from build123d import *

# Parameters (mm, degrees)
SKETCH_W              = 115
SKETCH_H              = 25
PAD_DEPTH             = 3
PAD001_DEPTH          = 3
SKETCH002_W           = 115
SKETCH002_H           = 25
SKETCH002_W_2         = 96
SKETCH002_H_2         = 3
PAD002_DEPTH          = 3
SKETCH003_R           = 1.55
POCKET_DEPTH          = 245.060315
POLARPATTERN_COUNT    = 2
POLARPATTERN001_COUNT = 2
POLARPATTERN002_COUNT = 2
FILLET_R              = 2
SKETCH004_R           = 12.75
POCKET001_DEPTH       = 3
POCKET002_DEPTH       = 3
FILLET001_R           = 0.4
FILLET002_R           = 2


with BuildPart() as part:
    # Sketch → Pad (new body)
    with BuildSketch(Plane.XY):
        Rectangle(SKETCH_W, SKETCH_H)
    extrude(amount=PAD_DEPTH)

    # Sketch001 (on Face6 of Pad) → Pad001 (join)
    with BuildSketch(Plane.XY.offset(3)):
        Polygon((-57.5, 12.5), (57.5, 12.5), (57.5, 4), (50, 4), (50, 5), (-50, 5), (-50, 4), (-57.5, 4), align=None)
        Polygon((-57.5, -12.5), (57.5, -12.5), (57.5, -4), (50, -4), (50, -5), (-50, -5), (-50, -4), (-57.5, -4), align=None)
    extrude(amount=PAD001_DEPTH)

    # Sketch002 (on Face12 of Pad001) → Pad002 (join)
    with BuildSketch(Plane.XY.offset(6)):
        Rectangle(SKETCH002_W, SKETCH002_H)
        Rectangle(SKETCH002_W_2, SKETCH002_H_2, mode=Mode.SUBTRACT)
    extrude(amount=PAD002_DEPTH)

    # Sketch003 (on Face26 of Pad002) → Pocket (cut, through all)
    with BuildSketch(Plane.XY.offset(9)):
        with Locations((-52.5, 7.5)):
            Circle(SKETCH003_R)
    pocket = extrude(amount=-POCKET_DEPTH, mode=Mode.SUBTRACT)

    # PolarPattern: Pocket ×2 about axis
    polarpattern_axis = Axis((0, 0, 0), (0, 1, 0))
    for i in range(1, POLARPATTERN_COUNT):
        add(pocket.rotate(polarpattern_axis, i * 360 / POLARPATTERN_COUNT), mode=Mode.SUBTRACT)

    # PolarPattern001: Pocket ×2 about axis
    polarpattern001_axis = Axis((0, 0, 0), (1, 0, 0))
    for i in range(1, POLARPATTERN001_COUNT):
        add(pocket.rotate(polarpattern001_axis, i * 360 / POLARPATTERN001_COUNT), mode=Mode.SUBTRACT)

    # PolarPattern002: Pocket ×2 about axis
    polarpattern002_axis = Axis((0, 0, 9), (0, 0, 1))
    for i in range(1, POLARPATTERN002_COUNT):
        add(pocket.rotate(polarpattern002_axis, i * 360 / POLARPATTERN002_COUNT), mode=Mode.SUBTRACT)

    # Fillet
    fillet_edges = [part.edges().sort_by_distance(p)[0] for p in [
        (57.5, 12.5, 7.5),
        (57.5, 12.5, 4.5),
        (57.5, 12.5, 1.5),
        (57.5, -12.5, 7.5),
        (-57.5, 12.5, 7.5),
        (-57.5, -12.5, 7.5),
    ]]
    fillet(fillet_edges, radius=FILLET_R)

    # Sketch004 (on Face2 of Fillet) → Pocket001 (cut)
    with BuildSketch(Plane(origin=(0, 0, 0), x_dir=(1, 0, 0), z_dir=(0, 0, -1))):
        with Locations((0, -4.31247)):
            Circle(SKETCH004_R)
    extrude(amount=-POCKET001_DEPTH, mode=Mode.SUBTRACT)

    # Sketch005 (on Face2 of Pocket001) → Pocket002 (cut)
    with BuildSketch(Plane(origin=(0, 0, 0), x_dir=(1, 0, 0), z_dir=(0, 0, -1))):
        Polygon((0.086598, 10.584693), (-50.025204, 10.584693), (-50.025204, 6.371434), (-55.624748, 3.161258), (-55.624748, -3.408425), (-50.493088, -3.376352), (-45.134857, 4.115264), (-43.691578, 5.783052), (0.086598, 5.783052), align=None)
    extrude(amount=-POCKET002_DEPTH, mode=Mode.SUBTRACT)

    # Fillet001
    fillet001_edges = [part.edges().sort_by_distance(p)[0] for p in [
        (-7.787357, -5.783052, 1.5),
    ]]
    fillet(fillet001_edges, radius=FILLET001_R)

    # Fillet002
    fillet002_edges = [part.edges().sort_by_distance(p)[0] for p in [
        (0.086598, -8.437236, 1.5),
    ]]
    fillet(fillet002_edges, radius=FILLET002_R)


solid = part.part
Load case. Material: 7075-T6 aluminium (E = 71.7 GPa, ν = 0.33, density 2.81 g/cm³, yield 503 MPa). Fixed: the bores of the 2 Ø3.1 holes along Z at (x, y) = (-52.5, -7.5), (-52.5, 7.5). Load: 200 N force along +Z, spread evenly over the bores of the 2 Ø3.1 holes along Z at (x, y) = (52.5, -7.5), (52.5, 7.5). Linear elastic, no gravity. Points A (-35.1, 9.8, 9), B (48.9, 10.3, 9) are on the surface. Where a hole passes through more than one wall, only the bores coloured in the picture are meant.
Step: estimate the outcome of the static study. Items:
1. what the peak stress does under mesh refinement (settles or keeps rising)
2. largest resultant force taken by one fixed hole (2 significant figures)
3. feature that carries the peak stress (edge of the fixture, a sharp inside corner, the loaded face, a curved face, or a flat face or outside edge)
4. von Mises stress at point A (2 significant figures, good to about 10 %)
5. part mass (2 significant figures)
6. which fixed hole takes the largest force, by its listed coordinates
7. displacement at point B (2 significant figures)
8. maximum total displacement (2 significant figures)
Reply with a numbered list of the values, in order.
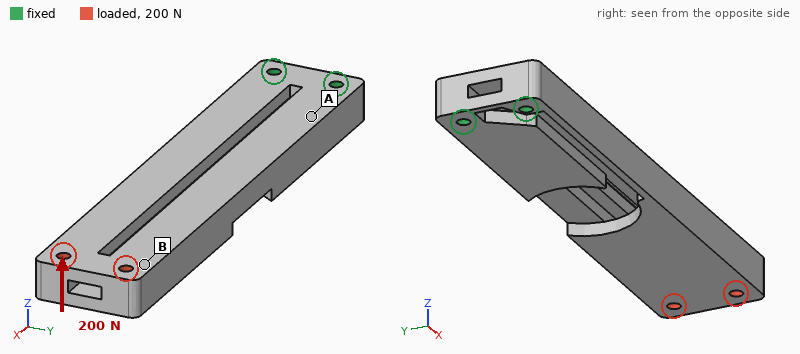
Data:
1. keeps rising
2. 300 N
3. a sharp inside corner
4. 65 MPa
5. 54 g
6. (-52.5, 7.5)
7. 1.2 mm
8. 1.4 mm
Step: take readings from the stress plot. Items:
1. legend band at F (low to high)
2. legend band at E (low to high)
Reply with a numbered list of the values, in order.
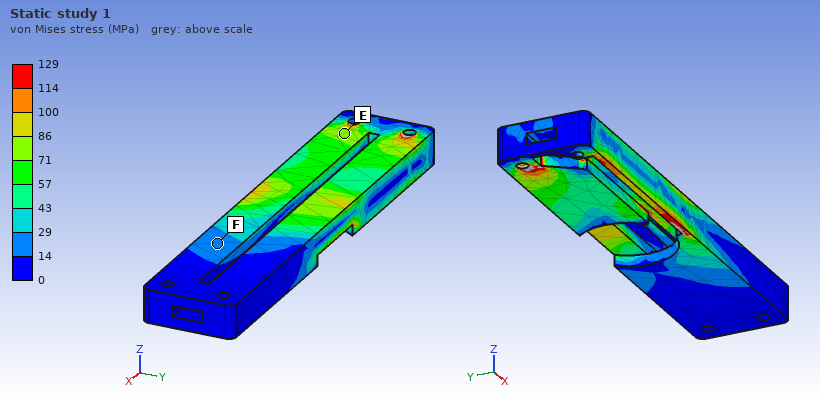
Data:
1. 14 to 29 MPa
2. 71 to 86 MPa
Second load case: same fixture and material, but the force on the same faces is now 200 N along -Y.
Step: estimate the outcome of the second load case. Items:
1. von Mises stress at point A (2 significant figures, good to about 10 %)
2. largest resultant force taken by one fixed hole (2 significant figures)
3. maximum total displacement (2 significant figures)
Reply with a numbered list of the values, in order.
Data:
1. 18 MPa
2. 1.2 kN
3. 0.18 mm
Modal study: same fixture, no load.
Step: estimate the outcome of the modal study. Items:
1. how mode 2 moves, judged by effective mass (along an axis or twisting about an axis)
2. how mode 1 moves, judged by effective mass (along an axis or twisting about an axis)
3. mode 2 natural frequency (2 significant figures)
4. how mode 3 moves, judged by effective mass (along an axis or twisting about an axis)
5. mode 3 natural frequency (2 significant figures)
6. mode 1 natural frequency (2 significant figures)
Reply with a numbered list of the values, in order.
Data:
1. along Y
2. along Z
3. 1400 Hz
4. twisting about X
5. 2500 Hz
6. 510 Hz
